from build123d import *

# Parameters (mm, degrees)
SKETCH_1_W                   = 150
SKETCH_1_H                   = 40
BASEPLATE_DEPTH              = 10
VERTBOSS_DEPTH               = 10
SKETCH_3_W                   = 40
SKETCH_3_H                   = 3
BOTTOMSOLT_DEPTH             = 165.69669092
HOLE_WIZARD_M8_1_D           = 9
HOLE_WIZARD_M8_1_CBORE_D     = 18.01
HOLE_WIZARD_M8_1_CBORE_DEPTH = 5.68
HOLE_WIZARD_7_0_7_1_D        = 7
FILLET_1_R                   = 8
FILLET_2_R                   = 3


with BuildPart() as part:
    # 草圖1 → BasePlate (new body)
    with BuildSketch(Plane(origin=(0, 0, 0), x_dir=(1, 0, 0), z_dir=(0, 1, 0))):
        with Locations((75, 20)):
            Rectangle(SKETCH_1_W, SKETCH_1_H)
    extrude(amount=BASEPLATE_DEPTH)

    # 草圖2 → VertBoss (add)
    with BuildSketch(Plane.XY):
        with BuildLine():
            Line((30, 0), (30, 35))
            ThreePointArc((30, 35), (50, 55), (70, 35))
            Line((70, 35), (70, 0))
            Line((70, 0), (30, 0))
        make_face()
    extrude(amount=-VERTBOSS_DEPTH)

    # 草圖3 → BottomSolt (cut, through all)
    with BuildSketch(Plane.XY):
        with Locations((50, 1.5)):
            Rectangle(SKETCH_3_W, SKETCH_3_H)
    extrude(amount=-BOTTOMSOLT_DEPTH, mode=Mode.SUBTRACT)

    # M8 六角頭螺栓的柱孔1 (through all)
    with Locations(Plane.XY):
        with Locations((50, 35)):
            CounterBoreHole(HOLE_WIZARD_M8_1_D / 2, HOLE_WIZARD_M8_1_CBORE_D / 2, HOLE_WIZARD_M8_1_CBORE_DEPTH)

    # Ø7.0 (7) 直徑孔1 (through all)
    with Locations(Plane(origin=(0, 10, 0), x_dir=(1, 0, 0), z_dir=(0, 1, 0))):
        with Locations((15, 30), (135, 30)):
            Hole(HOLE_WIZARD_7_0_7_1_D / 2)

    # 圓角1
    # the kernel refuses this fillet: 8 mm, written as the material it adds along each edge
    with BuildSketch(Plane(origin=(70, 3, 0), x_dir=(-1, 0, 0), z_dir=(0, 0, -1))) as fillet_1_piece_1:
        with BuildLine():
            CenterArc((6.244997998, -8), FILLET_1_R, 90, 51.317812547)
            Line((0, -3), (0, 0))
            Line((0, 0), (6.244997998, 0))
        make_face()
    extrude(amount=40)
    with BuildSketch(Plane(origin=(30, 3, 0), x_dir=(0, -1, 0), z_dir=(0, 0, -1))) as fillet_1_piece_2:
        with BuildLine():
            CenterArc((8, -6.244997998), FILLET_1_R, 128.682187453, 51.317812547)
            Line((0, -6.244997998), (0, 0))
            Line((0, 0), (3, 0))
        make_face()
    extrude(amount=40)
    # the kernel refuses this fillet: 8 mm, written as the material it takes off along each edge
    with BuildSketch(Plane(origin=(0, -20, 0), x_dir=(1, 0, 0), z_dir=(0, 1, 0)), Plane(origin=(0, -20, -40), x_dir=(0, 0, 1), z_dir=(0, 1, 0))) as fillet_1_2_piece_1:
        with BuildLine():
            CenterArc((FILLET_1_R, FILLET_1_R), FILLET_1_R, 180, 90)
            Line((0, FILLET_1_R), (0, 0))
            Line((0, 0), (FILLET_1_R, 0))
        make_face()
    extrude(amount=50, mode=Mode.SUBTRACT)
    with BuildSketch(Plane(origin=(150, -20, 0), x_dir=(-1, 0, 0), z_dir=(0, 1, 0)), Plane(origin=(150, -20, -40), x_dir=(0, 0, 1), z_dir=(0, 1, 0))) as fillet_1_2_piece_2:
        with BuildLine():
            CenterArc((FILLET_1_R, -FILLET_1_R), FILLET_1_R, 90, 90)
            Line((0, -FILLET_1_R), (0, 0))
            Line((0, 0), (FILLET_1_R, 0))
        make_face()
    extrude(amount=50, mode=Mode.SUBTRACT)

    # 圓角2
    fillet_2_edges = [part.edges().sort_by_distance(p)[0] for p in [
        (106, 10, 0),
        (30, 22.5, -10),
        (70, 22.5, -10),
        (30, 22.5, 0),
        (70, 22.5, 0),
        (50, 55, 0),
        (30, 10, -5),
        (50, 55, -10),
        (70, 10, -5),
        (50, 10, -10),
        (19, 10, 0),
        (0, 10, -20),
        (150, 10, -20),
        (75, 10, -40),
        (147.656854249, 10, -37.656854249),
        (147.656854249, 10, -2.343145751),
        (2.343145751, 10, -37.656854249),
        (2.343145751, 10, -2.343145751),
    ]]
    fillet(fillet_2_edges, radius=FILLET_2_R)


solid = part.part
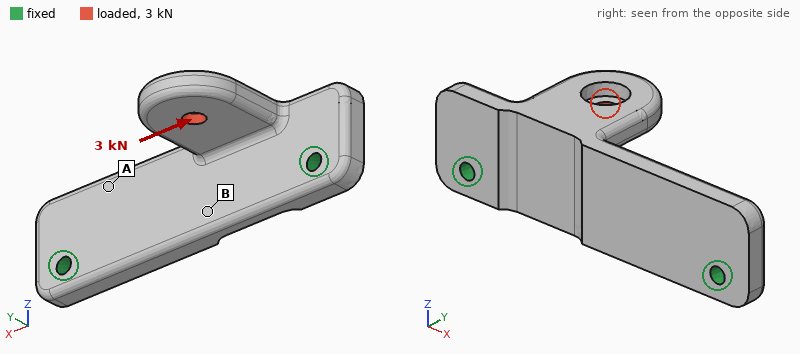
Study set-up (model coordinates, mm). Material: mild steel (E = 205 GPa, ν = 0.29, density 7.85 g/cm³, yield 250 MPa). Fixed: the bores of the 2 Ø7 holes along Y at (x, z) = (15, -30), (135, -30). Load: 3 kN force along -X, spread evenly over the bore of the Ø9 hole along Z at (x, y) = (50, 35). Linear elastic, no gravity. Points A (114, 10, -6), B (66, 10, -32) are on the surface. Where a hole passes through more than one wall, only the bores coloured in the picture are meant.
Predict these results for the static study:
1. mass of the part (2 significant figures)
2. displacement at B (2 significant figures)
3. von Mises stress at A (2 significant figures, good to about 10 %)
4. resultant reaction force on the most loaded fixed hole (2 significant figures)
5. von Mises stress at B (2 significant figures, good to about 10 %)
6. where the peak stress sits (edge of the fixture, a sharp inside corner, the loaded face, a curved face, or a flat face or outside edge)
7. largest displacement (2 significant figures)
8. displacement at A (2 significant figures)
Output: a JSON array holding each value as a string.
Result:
["530 g", "23 µm", "12 MPa", "1.9 kN", "35 MPa", "a curved face", "75 µm", "20 µm"]
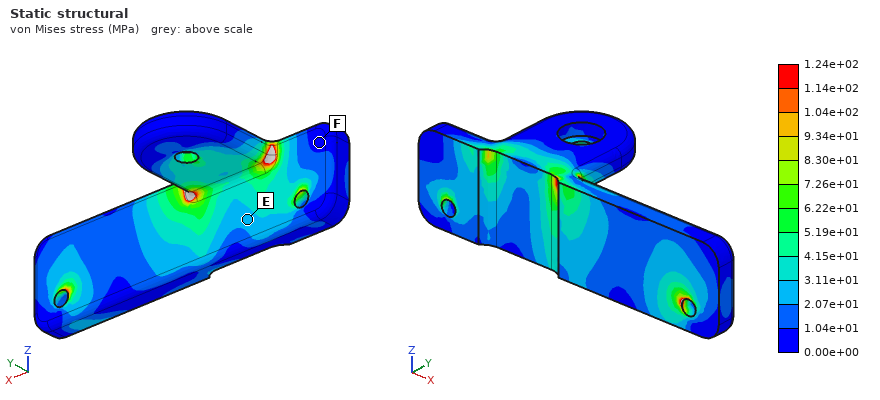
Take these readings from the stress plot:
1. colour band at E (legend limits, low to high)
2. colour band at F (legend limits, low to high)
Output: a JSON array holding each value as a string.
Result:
["2.07e+01 to 3.11e+01 MPa", "0.00e+00 to 1.04e+01 MPa"]
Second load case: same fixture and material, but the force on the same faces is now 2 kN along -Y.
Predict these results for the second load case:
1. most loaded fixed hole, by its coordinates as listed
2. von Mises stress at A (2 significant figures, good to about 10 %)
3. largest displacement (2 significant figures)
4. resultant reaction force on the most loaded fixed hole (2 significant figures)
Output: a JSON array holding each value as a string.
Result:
["(15, -30)", "14 MPa", "54 µm", "1.5 kN"]
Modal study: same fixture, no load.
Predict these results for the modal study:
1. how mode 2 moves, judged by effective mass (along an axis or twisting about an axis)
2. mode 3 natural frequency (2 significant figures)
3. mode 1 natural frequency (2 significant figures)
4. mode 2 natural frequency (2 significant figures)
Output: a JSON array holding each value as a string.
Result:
["along Y", "4900 Hz", "2000 Hz", "2700 Hz"]
